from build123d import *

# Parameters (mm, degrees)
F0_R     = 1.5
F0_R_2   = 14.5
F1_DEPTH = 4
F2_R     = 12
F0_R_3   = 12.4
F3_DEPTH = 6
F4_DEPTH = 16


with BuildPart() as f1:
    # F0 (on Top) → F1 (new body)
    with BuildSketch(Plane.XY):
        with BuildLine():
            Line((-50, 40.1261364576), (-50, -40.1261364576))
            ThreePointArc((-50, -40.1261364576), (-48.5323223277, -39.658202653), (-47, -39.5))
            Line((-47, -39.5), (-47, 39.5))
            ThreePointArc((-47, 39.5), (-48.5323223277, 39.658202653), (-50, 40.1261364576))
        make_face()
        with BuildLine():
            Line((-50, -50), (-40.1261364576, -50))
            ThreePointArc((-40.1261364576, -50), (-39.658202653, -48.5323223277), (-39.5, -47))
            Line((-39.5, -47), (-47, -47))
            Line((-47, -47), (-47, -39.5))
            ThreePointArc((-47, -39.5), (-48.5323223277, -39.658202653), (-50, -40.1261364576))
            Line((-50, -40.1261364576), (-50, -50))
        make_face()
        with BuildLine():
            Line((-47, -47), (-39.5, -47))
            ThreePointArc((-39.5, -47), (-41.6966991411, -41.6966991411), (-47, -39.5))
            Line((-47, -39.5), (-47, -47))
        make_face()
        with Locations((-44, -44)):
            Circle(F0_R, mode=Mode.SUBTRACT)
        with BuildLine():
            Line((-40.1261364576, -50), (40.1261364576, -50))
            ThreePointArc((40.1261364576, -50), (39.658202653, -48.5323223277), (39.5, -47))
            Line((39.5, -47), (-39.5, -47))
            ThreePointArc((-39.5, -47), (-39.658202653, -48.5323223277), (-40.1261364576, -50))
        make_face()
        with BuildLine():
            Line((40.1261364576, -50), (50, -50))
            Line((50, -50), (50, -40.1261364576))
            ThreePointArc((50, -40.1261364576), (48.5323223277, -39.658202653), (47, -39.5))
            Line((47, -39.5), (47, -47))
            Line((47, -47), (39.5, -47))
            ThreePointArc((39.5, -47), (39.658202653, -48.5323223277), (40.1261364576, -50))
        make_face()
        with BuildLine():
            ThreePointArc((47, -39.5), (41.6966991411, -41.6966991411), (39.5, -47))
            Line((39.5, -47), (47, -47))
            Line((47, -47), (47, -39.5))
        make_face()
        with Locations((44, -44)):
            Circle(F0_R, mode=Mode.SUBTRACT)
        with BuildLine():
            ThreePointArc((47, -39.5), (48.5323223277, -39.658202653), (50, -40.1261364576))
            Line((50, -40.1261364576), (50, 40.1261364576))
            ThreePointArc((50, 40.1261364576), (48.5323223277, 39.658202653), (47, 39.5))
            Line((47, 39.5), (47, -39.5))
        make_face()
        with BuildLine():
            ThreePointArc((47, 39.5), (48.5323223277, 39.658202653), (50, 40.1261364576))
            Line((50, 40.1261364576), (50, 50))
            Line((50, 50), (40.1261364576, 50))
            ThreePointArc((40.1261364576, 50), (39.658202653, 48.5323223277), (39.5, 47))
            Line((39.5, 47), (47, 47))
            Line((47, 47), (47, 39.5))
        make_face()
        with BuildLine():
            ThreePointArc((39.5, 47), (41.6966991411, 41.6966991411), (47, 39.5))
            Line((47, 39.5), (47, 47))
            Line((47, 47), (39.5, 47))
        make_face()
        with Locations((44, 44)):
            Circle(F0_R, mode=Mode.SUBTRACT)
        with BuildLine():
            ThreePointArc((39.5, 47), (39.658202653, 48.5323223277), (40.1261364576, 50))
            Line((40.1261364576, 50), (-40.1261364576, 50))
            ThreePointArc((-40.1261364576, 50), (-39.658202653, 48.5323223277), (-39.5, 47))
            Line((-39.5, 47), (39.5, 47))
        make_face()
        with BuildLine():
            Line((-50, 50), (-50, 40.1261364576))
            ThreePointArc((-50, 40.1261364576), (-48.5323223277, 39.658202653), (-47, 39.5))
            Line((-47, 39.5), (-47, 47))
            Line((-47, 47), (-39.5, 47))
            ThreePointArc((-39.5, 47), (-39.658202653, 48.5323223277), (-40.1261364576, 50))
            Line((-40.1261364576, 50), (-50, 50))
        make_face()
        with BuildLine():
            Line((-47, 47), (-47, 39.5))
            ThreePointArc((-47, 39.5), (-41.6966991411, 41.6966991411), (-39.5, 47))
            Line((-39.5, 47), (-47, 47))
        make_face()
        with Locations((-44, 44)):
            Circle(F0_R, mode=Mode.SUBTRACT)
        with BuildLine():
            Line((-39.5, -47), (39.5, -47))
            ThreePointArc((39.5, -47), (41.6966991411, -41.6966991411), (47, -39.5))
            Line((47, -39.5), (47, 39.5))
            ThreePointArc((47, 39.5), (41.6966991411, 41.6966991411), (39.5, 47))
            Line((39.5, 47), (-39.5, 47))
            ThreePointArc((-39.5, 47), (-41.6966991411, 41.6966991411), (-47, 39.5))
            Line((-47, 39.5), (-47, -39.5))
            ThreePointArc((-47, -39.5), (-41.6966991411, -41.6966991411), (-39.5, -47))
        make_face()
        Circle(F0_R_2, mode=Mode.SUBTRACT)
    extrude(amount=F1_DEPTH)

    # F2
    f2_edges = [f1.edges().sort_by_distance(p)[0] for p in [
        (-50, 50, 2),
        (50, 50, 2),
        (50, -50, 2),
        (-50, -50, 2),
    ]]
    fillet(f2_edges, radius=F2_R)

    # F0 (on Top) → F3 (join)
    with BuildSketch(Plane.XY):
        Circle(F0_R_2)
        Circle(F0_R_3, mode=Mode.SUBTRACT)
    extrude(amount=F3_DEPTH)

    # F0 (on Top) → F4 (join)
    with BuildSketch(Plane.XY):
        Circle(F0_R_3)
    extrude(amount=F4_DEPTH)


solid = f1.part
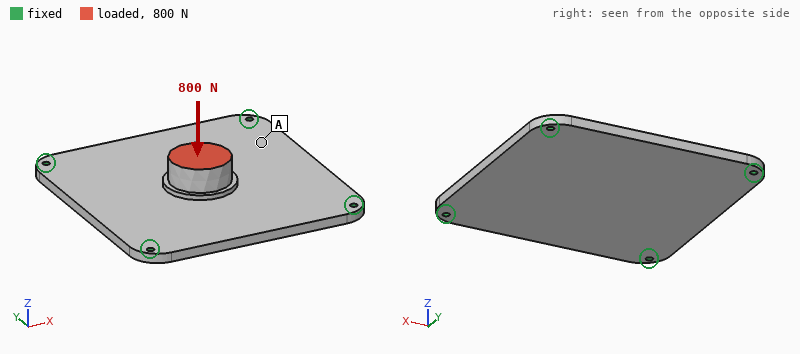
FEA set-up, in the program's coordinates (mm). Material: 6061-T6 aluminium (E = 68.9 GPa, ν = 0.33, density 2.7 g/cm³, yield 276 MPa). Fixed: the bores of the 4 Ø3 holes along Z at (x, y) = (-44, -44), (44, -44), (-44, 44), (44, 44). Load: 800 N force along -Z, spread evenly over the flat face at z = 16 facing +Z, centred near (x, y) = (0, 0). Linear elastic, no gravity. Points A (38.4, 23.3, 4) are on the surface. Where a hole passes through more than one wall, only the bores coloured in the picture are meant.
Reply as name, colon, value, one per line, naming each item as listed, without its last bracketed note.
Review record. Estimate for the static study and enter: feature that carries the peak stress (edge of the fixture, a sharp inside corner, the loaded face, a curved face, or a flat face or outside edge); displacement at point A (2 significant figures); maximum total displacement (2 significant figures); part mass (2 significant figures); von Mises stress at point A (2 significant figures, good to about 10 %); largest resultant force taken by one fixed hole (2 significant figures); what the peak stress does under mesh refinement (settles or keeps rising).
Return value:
feature that carries the peak stress: edge of the fixture
displacement at point A: 0.062 mm
maximum total displacement: 0.16 mm
part mass: 120 g
von Mises stress at point A: 8.1 MPa
largest resultant force taken by one fixed hole: 200 N
what the peak stress does under mesh refinement: keeps rising
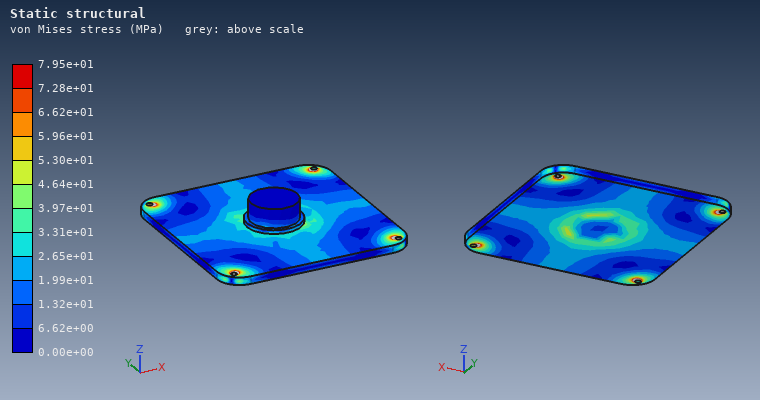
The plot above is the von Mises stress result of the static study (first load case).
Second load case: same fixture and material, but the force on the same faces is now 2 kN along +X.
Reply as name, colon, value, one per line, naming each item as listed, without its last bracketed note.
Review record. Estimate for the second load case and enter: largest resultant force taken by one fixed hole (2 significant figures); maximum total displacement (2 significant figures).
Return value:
largest resultant force taken by one fixed hole: 590 N
maximum total displacement: 0.11 mm
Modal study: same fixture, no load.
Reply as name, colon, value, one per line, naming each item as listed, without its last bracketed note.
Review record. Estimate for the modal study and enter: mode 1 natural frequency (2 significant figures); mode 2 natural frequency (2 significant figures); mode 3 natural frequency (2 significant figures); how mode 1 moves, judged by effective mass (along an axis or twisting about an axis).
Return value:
mode 1 natural frequency: 1400 Hz
mode 2 natural frequency: 2700 Hz
mode 3 natural frequency: 2700 Hz
how mode 1 moves, judged by effective mass: along Z
